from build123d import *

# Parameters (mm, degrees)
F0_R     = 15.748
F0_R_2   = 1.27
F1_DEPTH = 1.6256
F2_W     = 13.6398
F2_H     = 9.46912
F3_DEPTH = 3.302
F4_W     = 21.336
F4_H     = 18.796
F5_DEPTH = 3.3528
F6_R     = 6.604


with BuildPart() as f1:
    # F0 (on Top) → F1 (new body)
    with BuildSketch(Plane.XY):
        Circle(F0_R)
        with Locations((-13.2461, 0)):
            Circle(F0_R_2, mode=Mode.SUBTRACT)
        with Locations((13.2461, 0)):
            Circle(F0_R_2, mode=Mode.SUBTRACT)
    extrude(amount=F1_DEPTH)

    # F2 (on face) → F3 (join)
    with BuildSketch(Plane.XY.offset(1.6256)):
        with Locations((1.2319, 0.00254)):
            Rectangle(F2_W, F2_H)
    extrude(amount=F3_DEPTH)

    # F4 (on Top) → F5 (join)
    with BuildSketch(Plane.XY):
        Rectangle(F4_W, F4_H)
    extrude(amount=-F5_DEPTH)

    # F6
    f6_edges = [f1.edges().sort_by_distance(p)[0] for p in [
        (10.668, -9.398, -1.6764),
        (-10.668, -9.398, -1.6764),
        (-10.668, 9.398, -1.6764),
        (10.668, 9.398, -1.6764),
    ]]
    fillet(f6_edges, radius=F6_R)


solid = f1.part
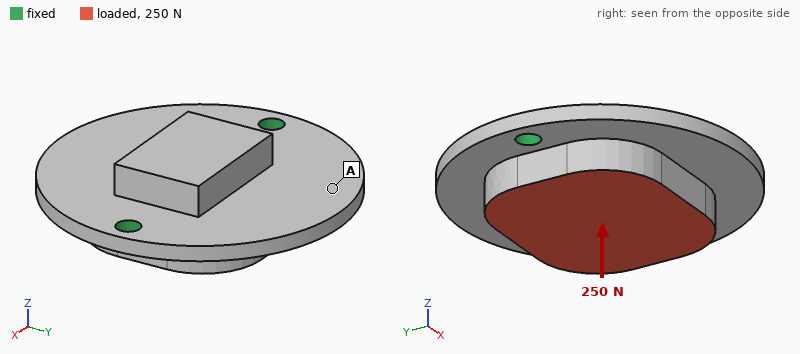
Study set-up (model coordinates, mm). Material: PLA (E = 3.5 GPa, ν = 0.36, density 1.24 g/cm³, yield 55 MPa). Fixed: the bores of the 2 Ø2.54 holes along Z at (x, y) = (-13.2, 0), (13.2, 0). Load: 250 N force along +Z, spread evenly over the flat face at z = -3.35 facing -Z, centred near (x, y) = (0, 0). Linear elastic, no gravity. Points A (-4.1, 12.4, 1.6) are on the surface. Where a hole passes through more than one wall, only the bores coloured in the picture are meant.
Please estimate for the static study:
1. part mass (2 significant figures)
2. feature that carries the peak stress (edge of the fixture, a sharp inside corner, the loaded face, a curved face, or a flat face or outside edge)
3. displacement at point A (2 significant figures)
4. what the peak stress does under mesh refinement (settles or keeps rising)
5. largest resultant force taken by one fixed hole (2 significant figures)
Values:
3.6 g
edge of the fixture
0.10 mm
keeps rising
140 N
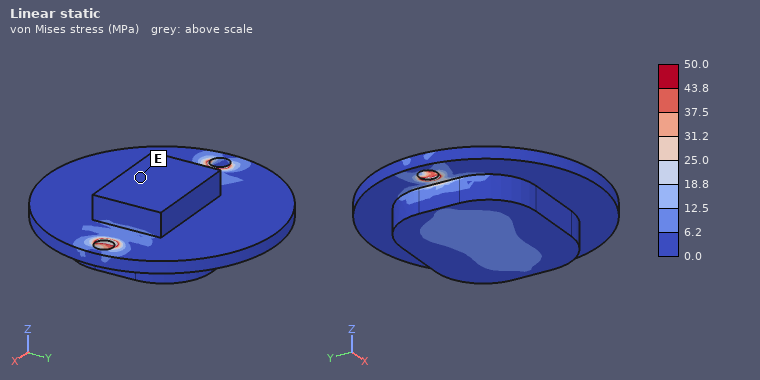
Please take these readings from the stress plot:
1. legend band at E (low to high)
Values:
0.0 to 6.2 MPa
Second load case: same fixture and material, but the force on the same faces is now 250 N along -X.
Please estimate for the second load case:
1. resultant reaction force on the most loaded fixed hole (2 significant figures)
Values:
130 N
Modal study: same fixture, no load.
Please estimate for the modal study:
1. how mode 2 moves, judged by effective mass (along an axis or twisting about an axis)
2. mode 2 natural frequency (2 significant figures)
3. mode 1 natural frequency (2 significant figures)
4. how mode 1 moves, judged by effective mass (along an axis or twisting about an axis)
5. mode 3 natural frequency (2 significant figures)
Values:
along Z
4600 Hz
1900 Hz
twisting about X
8600 Hz
